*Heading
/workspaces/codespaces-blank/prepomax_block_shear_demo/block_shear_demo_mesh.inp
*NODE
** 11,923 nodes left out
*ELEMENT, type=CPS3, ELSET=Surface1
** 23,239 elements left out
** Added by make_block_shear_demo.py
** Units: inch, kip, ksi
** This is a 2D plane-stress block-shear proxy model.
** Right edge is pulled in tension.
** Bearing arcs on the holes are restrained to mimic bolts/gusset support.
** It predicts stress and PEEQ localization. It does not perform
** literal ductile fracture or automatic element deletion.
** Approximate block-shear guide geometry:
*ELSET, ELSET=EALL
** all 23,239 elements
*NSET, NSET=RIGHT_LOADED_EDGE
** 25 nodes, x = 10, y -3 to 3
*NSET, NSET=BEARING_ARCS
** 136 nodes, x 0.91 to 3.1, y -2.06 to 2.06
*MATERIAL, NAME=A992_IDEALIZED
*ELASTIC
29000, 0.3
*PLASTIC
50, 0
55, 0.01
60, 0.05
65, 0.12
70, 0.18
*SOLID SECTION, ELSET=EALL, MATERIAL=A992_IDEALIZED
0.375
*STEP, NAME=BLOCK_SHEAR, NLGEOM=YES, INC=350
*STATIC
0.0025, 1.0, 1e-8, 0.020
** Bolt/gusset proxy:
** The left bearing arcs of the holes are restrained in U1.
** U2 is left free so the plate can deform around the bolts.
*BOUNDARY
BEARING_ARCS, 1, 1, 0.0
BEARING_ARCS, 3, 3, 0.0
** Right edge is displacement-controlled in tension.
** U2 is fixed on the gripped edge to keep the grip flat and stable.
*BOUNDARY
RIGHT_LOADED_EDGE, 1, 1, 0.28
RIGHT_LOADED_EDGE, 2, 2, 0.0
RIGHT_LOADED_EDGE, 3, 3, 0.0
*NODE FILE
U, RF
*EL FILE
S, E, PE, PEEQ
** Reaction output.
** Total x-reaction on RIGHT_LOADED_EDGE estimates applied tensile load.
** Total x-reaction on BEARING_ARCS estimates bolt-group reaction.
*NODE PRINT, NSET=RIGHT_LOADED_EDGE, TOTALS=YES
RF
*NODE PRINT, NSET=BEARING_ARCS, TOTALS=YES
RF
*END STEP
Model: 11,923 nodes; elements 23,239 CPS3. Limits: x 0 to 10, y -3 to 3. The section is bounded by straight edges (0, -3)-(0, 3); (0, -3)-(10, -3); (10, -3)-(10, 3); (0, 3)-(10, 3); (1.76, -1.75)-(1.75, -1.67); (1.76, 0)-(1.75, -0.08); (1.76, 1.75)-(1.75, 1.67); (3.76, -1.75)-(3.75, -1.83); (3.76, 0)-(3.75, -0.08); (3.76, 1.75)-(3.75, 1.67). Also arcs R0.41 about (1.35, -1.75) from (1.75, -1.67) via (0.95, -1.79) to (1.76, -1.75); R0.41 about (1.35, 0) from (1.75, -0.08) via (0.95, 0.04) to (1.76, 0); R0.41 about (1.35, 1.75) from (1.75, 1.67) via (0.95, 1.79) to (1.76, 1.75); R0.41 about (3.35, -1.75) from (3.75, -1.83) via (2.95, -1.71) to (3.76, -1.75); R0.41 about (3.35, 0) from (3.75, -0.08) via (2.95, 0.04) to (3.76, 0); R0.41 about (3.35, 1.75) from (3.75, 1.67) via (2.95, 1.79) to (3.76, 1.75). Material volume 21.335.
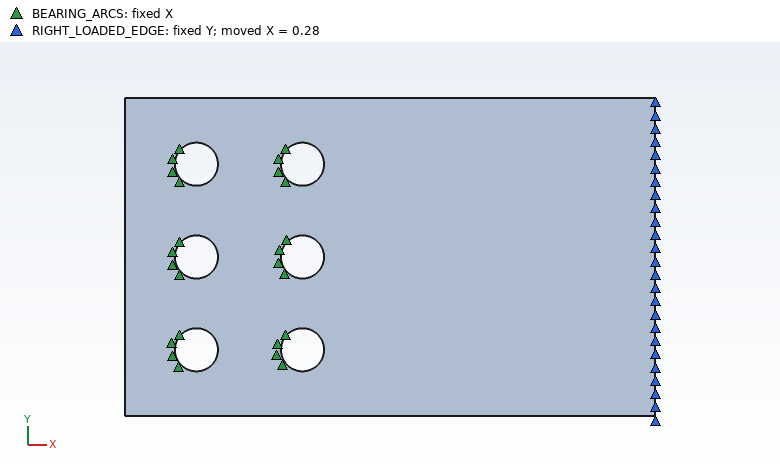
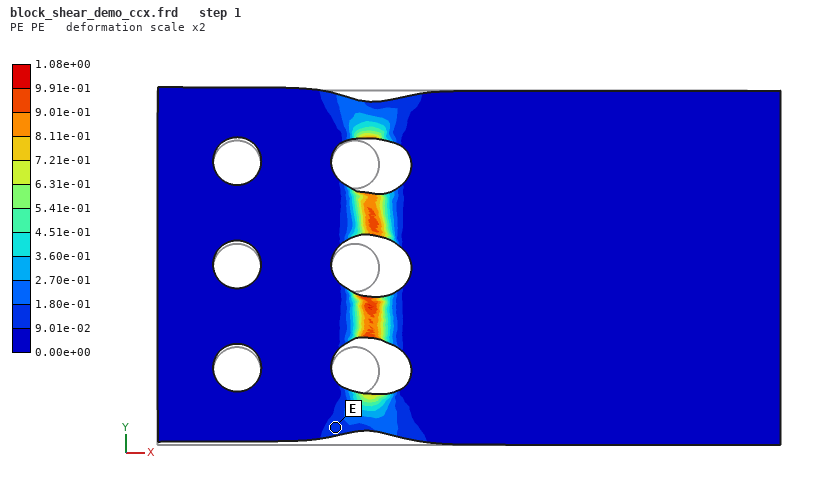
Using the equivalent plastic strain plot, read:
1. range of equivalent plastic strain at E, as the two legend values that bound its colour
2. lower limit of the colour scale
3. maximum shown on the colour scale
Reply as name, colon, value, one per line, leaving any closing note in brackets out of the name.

range of equivalent plastic strain at E, as the two legend values that bound its colour: 9.01e-02 to 1.80e-01
lower limit of the colour scale: 0.00e+00
maximum shown on the colour scale: 1.08e+00
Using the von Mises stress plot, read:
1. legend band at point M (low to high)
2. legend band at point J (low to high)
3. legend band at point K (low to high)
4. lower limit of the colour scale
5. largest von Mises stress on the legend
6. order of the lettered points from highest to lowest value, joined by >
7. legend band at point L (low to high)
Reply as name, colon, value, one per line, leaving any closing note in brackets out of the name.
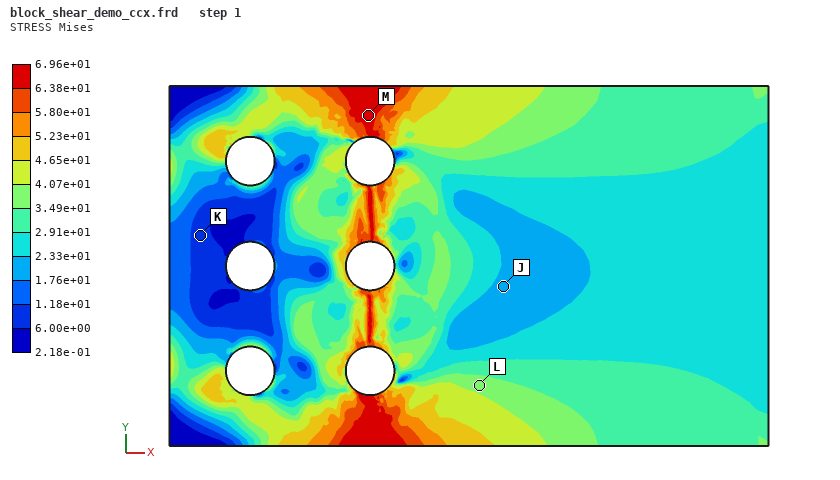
legend band at point M: 6.38e+01 to 6.96e+01
legend band at point J: 1.76e+01 to 2.33e+01
legend band at point K: 6.00e+00 to 1.18e+01
lower limit of the colour scale: 2.18e-01
largest von Mises stress on the legend: 6.96e+01
order of the lettered points from highest to lowest value, joined by >: M > L > J > K
legend band at point L: 3.49e+01 to 4.07e+01
